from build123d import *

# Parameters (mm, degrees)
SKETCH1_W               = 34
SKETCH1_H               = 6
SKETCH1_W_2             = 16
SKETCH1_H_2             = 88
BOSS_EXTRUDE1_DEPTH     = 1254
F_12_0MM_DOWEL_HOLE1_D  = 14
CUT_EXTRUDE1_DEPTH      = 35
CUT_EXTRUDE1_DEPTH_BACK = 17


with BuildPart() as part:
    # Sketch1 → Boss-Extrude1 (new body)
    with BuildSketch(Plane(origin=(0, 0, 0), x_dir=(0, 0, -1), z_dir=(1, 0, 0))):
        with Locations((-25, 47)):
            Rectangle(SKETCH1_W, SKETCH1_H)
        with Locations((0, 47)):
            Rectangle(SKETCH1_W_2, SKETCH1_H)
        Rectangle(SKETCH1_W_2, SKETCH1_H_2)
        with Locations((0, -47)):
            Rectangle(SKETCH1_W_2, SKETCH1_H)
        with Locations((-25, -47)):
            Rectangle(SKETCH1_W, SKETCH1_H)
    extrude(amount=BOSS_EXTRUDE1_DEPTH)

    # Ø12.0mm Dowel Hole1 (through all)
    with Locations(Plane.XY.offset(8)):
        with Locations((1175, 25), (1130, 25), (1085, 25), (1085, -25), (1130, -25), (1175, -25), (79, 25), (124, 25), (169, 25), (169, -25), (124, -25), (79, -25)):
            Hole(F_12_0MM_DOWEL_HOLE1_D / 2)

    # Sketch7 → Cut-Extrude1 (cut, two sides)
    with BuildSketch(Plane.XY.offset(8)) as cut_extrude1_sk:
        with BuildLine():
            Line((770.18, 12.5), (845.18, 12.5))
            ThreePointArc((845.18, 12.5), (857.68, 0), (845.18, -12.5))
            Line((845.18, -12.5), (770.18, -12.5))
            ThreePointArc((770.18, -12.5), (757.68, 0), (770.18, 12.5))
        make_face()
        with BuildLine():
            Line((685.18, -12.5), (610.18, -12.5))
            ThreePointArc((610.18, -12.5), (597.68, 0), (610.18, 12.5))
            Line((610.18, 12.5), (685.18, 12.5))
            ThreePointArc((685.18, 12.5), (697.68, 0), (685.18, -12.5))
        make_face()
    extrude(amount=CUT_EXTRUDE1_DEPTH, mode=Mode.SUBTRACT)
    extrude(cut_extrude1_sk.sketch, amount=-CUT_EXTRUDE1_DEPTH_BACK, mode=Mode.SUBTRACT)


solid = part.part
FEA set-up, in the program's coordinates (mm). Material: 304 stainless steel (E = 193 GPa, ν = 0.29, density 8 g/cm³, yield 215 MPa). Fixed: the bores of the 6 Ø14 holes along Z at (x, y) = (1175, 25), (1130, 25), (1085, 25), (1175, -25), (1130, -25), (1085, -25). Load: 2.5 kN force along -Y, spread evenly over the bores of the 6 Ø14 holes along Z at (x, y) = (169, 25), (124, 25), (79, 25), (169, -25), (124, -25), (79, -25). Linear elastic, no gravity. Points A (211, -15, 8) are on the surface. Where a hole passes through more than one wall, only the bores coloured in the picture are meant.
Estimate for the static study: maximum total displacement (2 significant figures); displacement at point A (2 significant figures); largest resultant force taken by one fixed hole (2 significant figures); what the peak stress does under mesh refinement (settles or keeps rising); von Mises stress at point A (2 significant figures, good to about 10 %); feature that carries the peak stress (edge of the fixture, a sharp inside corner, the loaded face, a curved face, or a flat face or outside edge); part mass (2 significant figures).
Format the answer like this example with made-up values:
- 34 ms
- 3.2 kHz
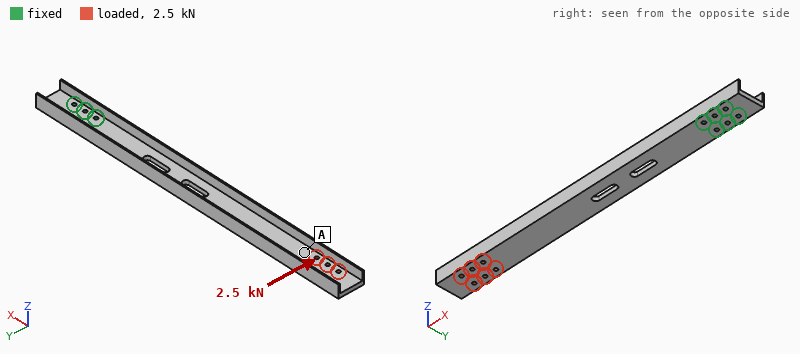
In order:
- 2.3 mm
- 1.7 mm
- 26 kN
- keeps rising
- 7.8 MPa
- edge of the fixture
- 19 kg
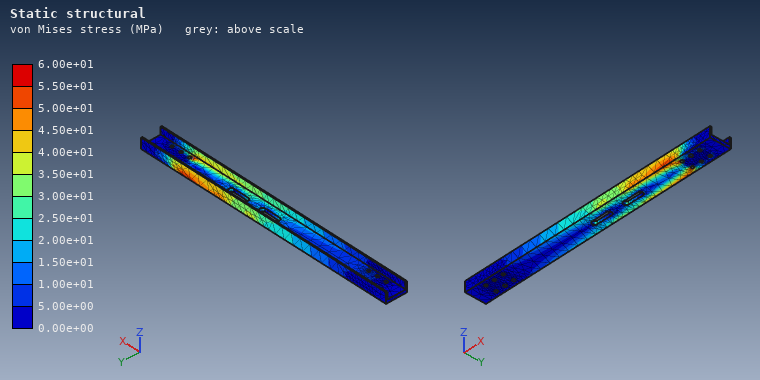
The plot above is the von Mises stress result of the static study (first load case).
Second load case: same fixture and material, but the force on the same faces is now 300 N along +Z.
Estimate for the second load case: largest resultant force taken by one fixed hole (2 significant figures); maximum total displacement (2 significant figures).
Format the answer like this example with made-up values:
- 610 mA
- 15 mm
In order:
- 2.3 kN
- 2.2 mm
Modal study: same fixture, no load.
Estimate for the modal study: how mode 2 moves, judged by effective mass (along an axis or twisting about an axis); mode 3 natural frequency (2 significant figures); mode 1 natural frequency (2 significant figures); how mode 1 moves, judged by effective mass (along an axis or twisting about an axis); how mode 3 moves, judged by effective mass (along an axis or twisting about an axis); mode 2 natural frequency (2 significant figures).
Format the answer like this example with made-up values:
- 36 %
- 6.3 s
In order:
- along Y
- 160 Hz
- 26 Hz
- along Z
- twisting about X
- 73 Hz
